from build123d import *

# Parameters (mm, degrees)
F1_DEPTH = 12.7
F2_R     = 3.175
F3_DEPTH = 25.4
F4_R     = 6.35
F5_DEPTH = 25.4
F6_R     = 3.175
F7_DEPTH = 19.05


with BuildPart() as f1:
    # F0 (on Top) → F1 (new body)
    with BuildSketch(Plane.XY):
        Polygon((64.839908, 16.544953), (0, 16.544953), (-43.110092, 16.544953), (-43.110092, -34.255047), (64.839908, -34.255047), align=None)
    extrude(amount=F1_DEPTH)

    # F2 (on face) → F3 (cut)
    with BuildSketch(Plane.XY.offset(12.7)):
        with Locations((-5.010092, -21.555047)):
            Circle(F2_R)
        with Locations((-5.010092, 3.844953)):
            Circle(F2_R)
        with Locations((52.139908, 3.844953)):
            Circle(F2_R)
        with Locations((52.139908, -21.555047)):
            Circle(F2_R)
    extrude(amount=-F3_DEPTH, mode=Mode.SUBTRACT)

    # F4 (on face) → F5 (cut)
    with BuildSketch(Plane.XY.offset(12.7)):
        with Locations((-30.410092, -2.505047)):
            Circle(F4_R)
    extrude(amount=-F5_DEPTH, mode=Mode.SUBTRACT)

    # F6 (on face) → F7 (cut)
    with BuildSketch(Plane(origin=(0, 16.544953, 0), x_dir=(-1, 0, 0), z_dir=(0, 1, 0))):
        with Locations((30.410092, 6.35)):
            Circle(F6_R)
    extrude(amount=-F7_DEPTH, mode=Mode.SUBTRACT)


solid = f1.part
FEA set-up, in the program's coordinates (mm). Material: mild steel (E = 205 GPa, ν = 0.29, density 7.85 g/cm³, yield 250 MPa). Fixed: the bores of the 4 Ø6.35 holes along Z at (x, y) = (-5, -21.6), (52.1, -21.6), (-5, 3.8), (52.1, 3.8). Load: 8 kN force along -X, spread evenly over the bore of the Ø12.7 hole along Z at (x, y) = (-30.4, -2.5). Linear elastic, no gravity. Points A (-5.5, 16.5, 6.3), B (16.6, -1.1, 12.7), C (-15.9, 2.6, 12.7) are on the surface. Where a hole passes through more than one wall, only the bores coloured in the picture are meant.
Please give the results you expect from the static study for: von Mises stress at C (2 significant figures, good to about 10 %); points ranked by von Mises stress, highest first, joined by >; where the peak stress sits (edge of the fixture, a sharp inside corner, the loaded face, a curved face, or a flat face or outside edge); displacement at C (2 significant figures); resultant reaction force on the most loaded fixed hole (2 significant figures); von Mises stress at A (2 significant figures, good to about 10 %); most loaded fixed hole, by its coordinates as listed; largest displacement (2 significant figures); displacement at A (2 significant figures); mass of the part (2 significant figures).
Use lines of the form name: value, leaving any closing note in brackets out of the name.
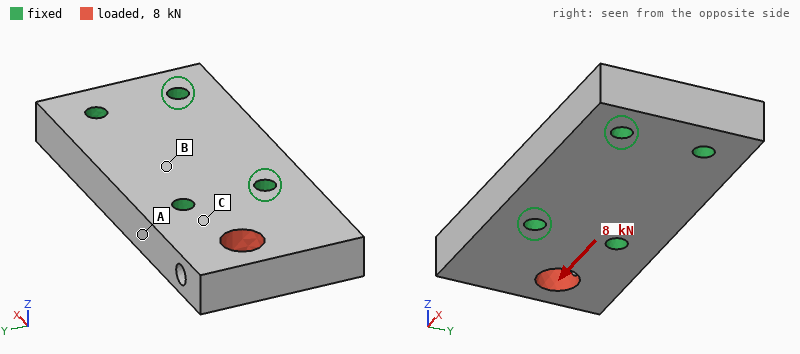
von Mises stress at C: 23 MPa
points ranked by von Mises stress, highest first, joined by >: C > A > B
where the peak stress sits: the loaded face
displacement at C: 1.1 µm
resultant reaction force on the most loaded fixed hole: 5.1 kN
von Mises stress at A: 13 MPa
most loaded fixed hole, by its coordinates as listed: (-5, 3.8)
largest displacement: 5.7 µm
displacement at A: 1.0 µm
mass of the part: 520 g
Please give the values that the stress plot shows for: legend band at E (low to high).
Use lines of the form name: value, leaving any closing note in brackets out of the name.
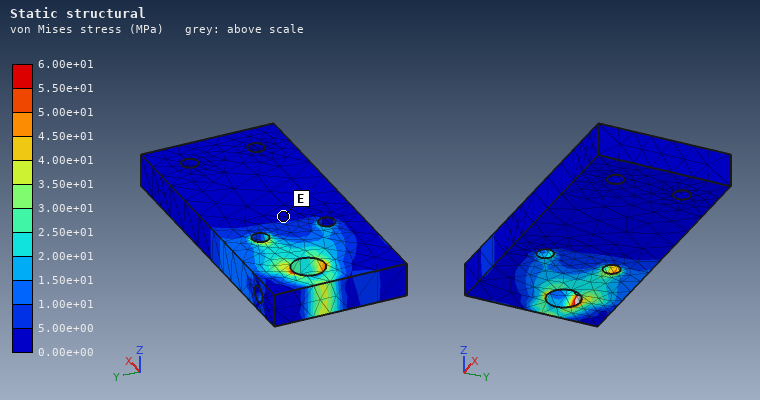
legend band at E: 0.00e+00 to 5.00e+00 MPa
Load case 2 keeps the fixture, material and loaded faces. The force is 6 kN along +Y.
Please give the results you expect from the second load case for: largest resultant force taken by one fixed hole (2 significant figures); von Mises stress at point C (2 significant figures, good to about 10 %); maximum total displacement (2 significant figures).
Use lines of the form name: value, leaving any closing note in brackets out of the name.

largest resultant force taken by one fixed hole: 5.1 kN
von Mises stress at point C: 22 MPa
maximum total displacement: 9.3 µm
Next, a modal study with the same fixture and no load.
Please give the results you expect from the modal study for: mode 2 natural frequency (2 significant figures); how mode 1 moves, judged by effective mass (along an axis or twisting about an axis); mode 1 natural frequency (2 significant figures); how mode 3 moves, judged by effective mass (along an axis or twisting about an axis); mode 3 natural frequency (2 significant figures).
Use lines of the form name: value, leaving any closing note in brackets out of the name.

mode 2 natural frequency: 11 kHz
how mode 1 moves, judged by effective mass: along Z
mode 1 natural frequency: 6800 Hz
how mode 3 moves, judged by effective mass: along Y
mode 3 natural frequency: 14 kHz
